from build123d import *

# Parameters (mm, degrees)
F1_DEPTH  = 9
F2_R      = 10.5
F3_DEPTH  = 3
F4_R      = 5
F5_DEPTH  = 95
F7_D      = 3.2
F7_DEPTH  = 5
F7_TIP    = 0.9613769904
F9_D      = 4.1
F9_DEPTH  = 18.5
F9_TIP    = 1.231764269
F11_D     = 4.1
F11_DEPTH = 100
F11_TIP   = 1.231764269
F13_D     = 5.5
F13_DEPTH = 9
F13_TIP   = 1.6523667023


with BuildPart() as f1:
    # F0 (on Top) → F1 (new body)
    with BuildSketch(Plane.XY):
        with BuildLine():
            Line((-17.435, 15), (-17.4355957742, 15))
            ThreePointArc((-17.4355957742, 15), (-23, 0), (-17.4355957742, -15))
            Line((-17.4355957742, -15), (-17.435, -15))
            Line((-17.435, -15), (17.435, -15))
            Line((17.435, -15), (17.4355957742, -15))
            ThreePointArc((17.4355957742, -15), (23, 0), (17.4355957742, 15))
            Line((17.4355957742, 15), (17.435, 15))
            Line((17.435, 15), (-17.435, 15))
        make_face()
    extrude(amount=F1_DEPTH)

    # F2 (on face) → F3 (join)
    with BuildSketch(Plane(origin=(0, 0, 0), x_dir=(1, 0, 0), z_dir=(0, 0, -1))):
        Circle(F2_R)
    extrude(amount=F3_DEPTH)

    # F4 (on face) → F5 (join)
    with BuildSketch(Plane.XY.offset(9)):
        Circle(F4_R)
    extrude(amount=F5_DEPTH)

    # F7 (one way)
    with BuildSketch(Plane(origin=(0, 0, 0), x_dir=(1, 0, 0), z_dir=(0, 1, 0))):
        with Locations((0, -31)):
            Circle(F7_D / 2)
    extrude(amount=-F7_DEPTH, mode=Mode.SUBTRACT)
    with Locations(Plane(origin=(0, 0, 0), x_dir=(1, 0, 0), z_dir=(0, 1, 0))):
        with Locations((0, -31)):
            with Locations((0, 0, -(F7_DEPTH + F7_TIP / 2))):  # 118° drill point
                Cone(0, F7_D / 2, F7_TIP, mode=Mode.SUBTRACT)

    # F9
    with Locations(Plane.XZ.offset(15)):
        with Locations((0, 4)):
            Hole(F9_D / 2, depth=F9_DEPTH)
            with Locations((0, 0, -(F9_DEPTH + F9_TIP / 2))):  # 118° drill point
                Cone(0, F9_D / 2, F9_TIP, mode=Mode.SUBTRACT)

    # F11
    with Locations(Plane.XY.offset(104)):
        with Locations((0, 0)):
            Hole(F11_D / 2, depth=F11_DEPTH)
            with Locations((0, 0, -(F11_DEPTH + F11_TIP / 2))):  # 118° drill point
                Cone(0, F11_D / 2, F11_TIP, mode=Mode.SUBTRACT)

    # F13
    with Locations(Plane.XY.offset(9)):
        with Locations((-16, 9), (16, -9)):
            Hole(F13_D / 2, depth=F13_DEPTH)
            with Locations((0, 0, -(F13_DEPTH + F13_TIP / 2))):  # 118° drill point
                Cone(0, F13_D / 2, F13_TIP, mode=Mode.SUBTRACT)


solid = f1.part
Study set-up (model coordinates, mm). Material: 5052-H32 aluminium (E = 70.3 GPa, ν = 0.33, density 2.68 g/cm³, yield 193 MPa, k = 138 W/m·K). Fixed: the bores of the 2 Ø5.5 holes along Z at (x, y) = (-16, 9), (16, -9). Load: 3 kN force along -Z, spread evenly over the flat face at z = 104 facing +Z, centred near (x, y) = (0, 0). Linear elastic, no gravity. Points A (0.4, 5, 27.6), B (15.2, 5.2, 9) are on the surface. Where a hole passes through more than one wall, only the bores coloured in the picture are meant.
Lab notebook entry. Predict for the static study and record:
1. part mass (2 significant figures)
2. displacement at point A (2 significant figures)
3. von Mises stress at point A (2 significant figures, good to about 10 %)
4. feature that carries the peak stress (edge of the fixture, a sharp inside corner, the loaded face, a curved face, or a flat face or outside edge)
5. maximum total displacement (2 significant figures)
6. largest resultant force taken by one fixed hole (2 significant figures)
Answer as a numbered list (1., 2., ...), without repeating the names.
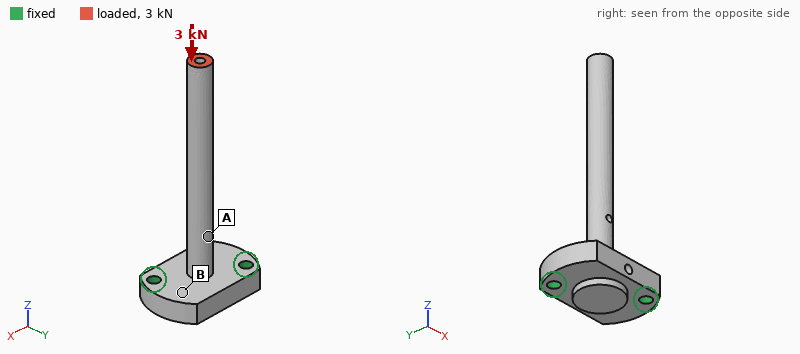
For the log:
1. 48 g
2. 22 µm
3. 41 MPa
4. a curved face
5. 83 µm
6. 1.5 kN
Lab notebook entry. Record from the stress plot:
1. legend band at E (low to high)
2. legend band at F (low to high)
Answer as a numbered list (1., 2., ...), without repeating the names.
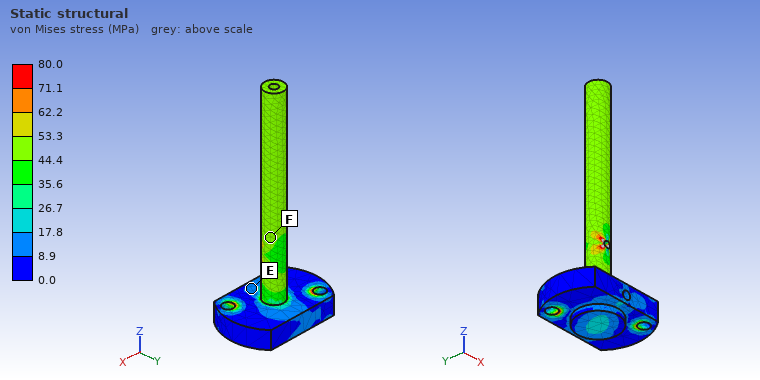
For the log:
1. 8.9 to 17.8 MPa
2. 44.4 to 53.3 MPa
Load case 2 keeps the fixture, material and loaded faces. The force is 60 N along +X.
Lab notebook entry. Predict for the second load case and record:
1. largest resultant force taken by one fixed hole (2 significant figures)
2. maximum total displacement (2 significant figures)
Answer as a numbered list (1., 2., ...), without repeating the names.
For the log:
1. 190 N
2. 0.57 mm
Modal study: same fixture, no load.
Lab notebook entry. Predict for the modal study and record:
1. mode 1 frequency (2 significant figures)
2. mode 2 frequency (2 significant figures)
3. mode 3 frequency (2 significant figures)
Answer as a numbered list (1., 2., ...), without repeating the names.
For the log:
1. 770 Hz
2. 800 Hz
3. 4700 Hz
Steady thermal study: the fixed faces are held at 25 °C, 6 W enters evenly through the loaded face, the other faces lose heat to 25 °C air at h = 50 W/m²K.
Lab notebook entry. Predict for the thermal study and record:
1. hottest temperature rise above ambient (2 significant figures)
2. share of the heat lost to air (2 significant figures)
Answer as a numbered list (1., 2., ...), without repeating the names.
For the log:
1. 39 K
2. 61 %
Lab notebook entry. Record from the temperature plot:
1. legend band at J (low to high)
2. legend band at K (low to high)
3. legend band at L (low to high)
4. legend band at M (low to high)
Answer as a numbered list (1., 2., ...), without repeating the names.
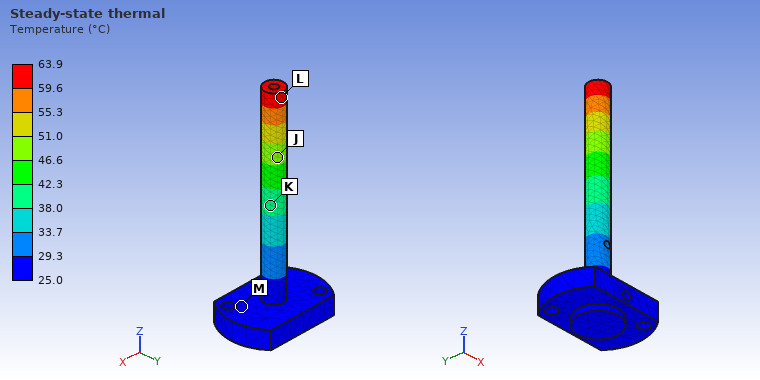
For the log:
1. 46.6 to 51.0 °C
2. 38.0 to 42.3 °C
3. 59.6 to 63.9 °C
4. 25.0 to 29.3 °C
